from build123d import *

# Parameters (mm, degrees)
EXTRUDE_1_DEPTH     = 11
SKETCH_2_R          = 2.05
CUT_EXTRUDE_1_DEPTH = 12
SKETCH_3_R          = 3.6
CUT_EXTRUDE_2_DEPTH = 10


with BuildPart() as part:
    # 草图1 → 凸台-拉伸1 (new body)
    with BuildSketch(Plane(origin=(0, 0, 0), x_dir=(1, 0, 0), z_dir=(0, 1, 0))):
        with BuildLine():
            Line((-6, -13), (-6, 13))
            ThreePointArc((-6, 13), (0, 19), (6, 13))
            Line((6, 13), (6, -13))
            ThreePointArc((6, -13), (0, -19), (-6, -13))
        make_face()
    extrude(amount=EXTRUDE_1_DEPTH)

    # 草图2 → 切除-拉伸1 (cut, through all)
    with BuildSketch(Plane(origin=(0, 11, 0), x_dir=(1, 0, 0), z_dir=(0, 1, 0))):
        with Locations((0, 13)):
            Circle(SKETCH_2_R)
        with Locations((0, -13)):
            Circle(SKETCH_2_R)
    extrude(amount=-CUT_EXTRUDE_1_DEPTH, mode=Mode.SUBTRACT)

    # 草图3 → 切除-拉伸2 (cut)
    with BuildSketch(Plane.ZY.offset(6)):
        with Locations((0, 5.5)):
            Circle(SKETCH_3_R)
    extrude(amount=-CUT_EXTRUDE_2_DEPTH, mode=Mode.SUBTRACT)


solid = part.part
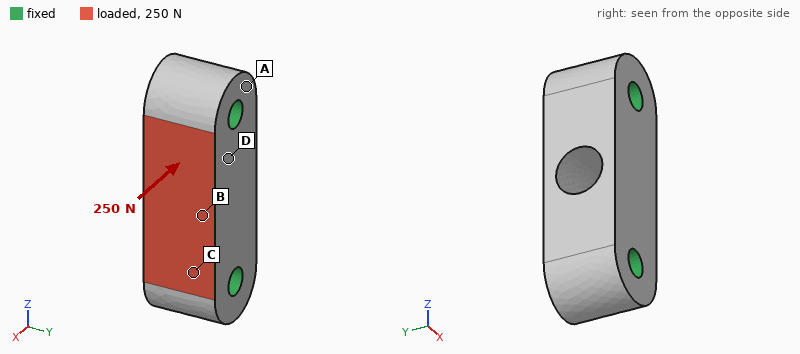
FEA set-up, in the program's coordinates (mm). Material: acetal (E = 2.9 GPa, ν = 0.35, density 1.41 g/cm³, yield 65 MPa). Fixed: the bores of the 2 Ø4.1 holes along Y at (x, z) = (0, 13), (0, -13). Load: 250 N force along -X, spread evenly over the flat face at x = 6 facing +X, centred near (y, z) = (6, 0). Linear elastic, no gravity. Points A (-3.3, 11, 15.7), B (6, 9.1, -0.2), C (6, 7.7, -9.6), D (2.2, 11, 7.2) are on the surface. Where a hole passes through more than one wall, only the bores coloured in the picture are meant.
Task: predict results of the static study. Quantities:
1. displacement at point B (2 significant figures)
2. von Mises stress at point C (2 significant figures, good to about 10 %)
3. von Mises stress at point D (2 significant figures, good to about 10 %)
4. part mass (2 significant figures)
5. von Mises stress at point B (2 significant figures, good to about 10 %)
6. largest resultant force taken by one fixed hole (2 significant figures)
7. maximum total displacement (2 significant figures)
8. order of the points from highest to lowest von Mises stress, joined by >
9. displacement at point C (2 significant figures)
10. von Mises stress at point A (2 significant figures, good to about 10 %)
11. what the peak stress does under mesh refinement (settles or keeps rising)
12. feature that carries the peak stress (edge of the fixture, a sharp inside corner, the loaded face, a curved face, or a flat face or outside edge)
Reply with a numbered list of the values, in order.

1. 13 µm
2. 0.99 MPa
3. 1.5 MPa
4. 5.6 g
5. 2.9 MPa
6. 130 N
7. 16 µm
8. B > D > C > A
9. 6.1 µm
10. 0.45 MPa
11. keeps rising
12. edge of the fixture
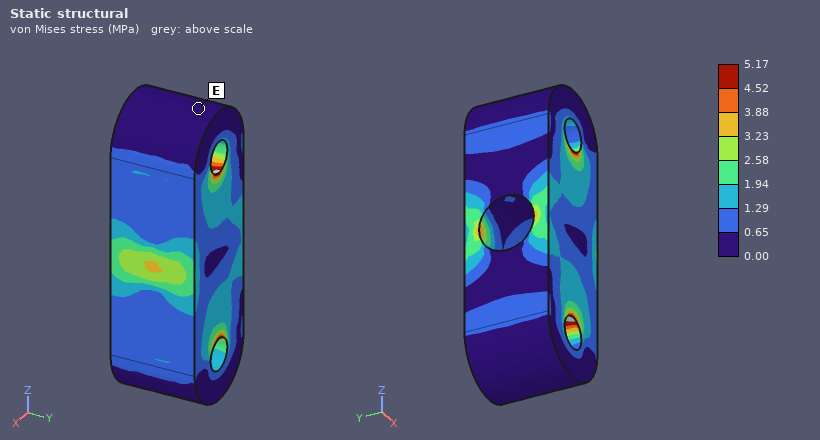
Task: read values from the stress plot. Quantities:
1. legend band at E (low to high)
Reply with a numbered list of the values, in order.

1. 0.00 to 0.65 MPa
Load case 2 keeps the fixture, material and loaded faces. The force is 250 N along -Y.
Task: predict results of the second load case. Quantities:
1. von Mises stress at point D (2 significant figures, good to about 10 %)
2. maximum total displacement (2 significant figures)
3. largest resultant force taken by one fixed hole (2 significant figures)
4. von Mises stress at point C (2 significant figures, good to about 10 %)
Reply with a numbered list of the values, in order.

1. 2.6 MPa
2. 28 µm
3. 130 N
4. 3.7 MPa
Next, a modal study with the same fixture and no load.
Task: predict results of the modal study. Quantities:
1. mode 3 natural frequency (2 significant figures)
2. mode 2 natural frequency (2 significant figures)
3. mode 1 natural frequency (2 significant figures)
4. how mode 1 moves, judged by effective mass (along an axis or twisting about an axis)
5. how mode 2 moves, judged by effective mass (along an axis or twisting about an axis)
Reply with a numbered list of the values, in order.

1. 17 kHz
2. 15 kHz
3. 13 kHz
4. along X
5. along Y
